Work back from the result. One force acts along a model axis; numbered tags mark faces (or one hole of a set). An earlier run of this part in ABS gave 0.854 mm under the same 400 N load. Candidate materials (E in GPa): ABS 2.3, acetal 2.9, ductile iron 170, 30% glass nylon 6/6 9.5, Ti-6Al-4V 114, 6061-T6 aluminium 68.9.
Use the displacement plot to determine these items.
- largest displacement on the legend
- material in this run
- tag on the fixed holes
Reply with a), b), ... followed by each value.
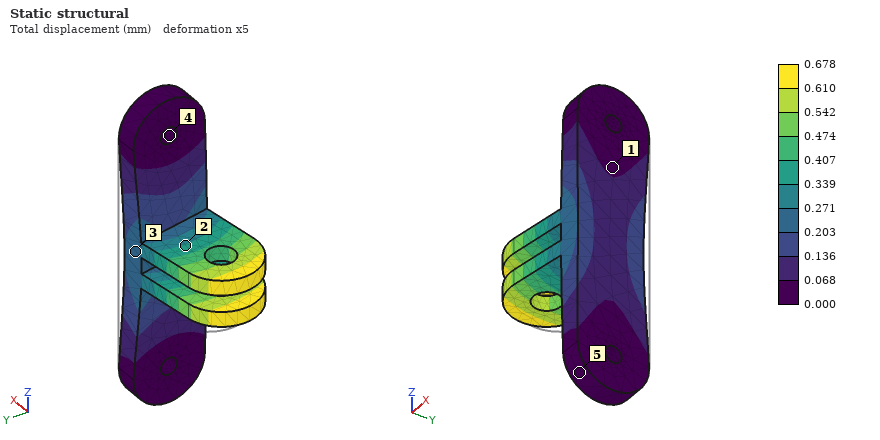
a) 0.678 mm
b) acetal
c) 4
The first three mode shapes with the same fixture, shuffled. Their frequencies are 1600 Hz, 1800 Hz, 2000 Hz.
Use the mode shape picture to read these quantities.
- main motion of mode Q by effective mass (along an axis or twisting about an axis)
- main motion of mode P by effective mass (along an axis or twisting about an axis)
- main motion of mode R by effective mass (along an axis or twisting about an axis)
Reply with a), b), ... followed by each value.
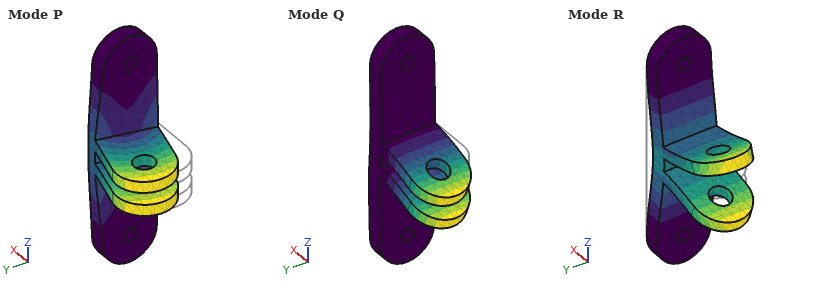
a) along Z
b) along Y
c) along X
